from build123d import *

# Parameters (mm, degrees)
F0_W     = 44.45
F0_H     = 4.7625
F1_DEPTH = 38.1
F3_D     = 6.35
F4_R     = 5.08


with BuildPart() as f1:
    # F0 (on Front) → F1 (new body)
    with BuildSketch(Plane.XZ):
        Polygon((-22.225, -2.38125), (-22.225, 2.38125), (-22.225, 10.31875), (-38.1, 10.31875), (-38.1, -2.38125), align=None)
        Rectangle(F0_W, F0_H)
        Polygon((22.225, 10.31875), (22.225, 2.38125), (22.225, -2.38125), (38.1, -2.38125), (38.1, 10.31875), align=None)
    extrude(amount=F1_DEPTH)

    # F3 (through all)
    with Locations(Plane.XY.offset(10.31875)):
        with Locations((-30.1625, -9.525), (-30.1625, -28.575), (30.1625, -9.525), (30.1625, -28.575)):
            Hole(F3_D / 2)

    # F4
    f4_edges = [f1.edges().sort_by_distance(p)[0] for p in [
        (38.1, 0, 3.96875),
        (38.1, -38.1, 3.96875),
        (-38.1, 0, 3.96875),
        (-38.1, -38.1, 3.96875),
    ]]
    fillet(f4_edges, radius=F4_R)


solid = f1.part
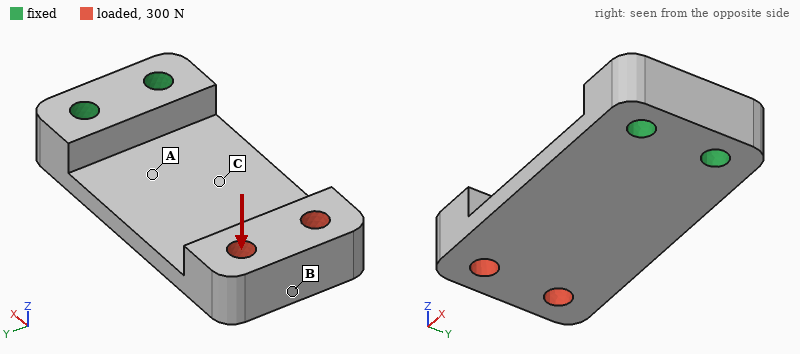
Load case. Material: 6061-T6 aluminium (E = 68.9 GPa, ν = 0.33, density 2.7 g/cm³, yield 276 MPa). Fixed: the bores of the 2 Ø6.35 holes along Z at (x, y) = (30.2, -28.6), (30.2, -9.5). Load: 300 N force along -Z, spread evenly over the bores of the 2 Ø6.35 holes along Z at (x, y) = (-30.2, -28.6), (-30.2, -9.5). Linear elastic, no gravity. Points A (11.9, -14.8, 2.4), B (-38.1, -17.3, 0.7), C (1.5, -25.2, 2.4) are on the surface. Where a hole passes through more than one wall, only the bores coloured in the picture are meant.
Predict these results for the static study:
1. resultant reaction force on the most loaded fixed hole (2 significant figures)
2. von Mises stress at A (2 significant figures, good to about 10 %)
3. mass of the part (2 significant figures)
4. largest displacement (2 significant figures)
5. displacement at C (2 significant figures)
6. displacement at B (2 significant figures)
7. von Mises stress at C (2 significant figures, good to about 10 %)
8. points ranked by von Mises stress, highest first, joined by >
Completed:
160 N
80 MPa
58 g
0.83 mm
0.16 mm
0.81 mm
61 MPa
A > C > B
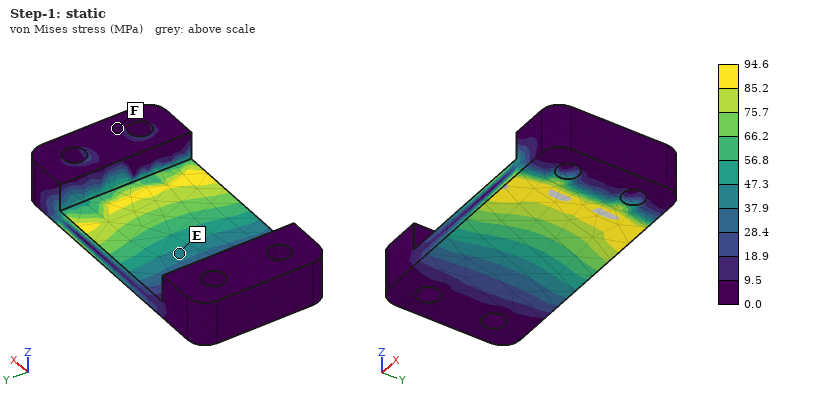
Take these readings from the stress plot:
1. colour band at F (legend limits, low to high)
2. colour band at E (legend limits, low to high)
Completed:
0.0 to 9.5 MPa
37.9 to 47.3 MPa
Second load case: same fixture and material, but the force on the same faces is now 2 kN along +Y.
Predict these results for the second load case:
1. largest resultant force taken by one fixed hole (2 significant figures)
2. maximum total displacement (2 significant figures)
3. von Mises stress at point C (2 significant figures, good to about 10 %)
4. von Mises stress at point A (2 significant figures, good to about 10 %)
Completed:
5.0 kN
0.28 mm
73 MPa
72 MPa
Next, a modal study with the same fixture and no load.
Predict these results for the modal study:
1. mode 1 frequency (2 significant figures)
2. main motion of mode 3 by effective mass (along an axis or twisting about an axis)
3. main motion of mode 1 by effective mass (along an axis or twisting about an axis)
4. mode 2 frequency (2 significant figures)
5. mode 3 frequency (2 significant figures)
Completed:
720 Hz
along Y
along Z
2600 Hz
4400 Hz
